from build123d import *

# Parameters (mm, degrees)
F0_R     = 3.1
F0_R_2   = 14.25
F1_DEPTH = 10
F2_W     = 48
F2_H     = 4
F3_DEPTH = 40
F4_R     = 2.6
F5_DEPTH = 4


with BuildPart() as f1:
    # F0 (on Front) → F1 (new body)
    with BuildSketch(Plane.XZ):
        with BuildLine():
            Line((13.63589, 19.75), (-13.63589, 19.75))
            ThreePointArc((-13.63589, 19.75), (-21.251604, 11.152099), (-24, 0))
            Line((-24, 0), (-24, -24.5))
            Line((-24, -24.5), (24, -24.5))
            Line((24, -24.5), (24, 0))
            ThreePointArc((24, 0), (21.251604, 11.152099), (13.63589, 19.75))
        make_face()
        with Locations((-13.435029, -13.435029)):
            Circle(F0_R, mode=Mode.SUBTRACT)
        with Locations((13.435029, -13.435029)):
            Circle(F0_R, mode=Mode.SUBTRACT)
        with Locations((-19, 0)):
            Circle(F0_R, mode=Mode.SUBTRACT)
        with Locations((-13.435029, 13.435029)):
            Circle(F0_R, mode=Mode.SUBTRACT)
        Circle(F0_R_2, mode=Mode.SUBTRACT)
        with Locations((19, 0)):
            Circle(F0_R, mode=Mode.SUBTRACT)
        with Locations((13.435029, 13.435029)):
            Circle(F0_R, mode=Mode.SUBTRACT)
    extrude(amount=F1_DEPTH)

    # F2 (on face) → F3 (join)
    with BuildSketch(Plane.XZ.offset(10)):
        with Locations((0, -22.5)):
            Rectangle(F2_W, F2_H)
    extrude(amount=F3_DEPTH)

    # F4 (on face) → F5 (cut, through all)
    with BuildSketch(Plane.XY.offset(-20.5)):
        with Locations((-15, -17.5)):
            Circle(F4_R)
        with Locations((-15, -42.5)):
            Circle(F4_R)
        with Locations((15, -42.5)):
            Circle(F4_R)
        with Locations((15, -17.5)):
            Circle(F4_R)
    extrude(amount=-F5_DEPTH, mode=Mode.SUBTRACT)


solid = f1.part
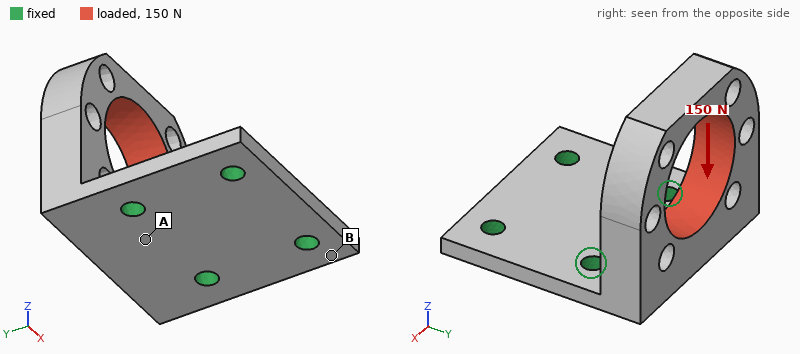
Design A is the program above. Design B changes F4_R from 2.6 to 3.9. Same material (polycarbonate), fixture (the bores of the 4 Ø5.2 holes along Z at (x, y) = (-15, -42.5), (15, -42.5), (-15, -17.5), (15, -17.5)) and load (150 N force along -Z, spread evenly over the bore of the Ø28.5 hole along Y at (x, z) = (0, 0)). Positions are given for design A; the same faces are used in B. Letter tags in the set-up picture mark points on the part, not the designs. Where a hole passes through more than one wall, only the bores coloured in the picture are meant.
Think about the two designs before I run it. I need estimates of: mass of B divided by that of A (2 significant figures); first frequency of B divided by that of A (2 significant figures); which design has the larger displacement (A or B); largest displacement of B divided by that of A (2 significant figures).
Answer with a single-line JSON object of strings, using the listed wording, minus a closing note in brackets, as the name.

{"mass of B divided by that of A": "0.98", "first frequency of B divided by that of A": "1.1", "which design has the larger displacement": "A", "largest displacement of B divided by that of A": "0.72"}
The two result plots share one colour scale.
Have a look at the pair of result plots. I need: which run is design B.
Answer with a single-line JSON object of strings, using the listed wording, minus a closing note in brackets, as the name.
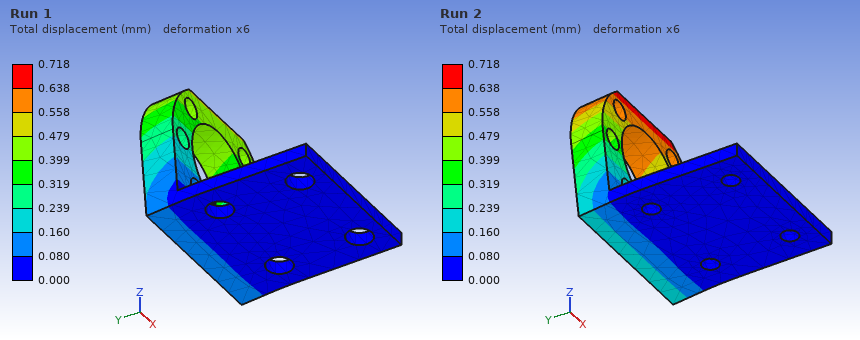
{"which run is design B": "Run 1"}
